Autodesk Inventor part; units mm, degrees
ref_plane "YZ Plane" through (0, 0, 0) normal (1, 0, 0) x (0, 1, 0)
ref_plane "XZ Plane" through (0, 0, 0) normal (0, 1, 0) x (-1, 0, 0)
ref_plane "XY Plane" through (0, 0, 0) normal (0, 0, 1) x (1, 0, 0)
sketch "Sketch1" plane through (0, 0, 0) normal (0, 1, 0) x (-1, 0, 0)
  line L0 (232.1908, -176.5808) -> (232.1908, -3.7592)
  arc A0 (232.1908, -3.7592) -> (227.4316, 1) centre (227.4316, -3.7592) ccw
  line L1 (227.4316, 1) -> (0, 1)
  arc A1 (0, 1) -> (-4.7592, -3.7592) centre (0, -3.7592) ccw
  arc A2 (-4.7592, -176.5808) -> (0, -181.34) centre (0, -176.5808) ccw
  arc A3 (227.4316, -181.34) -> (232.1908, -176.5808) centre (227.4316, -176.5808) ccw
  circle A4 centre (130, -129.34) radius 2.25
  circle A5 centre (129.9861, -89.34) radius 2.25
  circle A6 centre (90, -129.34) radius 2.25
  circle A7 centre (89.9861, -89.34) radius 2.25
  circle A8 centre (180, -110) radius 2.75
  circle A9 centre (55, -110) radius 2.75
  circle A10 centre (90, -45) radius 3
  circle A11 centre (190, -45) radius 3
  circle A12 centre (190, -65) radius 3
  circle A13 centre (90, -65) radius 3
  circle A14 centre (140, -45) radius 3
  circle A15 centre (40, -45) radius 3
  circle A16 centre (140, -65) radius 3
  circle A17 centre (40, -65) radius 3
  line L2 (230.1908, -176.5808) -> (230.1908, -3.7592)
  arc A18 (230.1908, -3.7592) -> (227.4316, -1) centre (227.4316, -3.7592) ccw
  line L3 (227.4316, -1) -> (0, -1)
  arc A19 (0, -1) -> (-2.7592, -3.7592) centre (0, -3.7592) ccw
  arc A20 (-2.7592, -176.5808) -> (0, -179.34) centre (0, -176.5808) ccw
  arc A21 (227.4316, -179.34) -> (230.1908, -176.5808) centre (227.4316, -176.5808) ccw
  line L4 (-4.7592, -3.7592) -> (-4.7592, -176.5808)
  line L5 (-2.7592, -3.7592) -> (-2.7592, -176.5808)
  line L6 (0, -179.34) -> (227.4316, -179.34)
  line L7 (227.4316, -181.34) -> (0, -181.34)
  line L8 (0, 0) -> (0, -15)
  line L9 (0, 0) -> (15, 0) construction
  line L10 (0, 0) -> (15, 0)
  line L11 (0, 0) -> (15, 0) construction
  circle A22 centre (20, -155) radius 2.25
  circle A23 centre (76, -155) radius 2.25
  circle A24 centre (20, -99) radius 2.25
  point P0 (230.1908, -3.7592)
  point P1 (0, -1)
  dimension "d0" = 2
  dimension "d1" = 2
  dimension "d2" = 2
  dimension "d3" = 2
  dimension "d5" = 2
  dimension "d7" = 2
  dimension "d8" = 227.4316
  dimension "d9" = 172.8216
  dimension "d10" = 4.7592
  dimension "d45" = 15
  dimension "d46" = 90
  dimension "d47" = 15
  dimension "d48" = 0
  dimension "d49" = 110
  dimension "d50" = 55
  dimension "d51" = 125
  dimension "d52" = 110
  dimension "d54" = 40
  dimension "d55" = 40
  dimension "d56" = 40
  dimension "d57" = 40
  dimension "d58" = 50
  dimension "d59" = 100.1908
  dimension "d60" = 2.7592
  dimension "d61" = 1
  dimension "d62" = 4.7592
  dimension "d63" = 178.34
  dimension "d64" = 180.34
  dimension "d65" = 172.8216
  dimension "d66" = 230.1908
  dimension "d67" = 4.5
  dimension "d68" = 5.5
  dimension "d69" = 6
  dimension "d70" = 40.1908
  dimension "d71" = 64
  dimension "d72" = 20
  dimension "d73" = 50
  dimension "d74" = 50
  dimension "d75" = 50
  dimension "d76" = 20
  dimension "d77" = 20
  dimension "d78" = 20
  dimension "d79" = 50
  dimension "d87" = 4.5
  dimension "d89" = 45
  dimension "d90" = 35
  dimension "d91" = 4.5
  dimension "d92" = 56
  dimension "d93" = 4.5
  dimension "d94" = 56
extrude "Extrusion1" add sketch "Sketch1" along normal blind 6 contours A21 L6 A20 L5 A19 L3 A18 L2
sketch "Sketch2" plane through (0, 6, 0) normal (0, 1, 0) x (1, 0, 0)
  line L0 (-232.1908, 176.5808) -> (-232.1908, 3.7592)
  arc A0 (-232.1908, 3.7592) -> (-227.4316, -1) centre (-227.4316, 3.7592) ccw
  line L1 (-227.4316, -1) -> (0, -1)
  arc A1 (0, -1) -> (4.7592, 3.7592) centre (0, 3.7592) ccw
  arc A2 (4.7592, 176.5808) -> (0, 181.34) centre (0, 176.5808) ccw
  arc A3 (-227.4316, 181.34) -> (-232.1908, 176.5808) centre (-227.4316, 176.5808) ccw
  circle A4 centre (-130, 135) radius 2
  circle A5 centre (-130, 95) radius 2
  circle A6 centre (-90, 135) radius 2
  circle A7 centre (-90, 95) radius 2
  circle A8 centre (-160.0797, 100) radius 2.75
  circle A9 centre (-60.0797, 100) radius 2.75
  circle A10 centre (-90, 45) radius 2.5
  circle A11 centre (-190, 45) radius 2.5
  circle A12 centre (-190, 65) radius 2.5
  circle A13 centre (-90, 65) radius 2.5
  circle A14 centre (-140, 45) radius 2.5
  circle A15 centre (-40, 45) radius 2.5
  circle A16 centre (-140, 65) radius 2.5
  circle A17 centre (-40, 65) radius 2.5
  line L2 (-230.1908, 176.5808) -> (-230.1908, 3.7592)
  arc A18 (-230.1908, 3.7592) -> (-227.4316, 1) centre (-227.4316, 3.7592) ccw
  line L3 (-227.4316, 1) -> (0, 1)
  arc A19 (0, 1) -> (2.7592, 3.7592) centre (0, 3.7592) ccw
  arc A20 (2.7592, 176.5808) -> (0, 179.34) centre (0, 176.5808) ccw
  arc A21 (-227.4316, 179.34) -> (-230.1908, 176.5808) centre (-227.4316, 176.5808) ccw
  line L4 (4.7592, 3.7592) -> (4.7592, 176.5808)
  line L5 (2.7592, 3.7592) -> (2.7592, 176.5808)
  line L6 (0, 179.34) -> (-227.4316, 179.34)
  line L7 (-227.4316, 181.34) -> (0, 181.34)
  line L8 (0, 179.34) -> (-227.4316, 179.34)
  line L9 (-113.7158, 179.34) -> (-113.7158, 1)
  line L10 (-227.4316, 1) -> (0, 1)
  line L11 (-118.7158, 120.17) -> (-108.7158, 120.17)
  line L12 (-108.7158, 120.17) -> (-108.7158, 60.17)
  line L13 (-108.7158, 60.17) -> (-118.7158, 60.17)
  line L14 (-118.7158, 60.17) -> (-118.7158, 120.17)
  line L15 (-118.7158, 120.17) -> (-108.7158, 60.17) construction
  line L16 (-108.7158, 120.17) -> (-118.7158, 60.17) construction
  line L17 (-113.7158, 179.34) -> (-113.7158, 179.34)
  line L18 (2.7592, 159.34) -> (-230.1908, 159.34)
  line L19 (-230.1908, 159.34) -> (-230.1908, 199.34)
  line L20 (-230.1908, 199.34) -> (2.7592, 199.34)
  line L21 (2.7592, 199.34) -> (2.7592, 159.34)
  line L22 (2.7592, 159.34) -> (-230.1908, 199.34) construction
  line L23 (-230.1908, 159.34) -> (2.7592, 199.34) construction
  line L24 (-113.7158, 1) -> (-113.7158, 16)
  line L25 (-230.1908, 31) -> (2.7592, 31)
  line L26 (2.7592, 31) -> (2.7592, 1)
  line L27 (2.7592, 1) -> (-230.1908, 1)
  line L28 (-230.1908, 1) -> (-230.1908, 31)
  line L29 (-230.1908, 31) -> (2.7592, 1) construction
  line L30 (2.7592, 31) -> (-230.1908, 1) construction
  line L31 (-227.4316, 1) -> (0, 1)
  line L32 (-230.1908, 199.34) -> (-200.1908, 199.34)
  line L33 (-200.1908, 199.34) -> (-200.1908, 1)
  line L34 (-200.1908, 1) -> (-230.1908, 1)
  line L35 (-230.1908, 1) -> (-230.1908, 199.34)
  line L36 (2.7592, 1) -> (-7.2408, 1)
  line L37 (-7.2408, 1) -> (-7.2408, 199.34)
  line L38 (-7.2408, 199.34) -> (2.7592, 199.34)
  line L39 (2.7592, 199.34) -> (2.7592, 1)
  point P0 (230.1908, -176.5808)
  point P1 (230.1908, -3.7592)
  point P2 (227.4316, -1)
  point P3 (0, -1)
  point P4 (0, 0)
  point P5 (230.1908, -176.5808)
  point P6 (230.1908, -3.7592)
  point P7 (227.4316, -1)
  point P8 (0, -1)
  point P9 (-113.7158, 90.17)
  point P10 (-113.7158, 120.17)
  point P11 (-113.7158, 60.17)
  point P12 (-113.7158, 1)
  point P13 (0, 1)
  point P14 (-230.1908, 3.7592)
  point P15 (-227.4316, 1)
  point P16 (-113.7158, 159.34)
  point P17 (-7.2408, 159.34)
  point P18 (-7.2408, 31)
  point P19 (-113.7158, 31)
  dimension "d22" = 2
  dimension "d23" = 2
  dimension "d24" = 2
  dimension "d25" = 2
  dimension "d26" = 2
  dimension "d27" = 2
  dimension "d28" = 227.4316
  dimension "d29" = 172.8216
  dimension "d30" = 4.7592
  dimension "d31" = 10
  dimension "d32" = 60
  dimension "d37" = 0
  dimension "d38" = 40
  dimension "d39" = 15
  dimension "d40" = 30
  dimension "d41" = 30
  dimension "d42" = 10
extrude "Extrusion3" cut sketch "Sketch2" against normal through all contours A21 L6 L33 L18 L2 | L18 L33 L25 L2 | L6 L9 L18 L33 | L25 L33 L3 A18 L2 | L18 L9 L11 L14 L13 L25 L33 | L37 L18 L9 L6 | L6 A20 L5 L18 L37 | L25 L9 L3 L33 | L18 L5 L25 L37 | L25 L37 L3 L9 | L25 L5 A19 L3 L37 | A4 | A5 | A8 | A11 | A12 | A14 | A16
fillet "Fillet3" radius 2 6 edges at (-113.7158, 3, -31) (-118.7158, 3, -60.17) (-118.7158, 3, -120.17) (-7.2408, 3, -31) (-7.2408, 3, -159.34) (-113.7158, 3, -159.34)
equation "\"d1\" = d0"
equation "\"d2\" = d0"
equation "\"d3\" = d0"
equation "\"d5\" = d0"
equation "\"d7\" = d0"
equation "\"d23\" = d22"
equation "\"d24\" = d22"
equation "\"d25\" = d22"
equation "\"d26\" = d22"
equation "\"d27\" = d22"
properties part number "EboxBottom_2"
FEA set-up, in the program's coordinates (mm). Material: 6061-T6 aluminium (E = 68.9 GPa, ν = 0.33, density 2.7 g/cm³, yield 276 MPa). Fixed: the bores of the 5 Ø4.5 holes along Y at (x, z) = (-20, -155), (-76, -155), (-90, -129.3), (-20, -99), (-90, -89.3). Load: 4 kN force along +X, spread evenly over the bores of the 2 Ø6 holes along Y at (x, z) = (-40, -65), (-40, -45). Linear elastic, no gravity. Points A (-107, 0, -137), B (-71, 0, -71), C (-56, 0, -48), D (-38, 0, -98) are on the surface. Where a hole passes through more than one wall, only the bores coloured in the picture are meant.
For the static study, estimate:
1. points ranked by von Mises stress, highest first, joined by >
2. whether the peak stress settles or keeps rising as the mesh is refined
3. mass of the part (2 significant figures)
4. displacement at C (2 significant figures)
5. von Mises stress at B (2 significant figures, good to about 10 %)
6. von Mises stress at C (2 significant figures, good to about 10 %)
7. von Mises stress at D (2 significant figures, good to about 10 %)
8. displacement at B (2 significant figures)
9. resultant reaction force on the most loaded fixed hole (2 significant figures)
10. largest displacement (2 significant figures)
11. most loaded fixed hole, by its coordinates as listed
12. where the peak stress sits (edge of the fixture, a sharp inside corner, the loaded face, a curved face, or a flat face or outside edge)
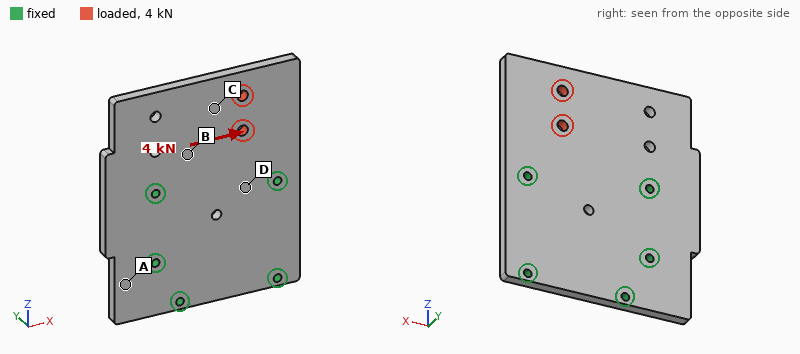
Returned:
B > C > D > A
keeps rising
220 g
17 µm
14 MPa
11 MPa
6.6 MPa
8.7 µm
2.8 kN
23 µm
(-90, -89.3)
edge of the fixture
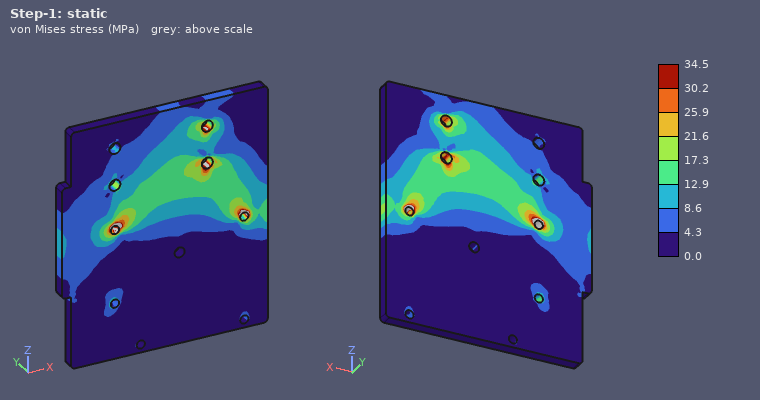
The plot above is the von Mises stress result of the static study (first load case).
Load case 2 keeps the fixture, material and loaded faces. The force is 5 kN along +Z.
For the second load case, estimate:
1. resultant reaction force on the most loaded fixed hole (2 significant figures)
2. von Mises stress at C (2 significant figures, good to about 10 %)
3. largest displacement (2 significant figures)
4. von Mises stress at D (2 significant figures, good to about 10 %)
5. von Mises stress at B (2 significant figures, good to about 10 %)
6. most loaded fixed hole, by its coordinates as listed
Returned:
2.8 kN
8.8 MPa
16 µm
8.2 MPa
5.9 MPa
(-20, -99)
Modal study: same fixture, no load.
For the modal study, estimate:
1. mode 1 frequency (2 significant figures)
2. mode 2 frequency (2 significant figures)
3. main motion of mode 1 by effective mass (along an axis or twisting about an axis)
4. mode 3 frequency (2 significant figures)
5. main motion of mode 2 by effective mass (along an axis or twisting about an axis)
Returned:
1100 Hz
2000 Hz
along Y
3700 Hz
twisting about Z
